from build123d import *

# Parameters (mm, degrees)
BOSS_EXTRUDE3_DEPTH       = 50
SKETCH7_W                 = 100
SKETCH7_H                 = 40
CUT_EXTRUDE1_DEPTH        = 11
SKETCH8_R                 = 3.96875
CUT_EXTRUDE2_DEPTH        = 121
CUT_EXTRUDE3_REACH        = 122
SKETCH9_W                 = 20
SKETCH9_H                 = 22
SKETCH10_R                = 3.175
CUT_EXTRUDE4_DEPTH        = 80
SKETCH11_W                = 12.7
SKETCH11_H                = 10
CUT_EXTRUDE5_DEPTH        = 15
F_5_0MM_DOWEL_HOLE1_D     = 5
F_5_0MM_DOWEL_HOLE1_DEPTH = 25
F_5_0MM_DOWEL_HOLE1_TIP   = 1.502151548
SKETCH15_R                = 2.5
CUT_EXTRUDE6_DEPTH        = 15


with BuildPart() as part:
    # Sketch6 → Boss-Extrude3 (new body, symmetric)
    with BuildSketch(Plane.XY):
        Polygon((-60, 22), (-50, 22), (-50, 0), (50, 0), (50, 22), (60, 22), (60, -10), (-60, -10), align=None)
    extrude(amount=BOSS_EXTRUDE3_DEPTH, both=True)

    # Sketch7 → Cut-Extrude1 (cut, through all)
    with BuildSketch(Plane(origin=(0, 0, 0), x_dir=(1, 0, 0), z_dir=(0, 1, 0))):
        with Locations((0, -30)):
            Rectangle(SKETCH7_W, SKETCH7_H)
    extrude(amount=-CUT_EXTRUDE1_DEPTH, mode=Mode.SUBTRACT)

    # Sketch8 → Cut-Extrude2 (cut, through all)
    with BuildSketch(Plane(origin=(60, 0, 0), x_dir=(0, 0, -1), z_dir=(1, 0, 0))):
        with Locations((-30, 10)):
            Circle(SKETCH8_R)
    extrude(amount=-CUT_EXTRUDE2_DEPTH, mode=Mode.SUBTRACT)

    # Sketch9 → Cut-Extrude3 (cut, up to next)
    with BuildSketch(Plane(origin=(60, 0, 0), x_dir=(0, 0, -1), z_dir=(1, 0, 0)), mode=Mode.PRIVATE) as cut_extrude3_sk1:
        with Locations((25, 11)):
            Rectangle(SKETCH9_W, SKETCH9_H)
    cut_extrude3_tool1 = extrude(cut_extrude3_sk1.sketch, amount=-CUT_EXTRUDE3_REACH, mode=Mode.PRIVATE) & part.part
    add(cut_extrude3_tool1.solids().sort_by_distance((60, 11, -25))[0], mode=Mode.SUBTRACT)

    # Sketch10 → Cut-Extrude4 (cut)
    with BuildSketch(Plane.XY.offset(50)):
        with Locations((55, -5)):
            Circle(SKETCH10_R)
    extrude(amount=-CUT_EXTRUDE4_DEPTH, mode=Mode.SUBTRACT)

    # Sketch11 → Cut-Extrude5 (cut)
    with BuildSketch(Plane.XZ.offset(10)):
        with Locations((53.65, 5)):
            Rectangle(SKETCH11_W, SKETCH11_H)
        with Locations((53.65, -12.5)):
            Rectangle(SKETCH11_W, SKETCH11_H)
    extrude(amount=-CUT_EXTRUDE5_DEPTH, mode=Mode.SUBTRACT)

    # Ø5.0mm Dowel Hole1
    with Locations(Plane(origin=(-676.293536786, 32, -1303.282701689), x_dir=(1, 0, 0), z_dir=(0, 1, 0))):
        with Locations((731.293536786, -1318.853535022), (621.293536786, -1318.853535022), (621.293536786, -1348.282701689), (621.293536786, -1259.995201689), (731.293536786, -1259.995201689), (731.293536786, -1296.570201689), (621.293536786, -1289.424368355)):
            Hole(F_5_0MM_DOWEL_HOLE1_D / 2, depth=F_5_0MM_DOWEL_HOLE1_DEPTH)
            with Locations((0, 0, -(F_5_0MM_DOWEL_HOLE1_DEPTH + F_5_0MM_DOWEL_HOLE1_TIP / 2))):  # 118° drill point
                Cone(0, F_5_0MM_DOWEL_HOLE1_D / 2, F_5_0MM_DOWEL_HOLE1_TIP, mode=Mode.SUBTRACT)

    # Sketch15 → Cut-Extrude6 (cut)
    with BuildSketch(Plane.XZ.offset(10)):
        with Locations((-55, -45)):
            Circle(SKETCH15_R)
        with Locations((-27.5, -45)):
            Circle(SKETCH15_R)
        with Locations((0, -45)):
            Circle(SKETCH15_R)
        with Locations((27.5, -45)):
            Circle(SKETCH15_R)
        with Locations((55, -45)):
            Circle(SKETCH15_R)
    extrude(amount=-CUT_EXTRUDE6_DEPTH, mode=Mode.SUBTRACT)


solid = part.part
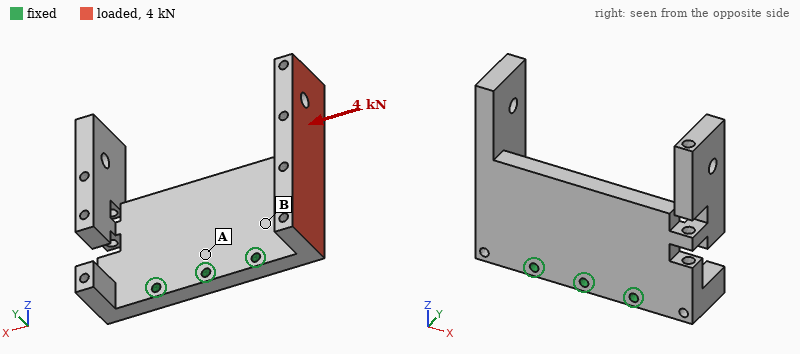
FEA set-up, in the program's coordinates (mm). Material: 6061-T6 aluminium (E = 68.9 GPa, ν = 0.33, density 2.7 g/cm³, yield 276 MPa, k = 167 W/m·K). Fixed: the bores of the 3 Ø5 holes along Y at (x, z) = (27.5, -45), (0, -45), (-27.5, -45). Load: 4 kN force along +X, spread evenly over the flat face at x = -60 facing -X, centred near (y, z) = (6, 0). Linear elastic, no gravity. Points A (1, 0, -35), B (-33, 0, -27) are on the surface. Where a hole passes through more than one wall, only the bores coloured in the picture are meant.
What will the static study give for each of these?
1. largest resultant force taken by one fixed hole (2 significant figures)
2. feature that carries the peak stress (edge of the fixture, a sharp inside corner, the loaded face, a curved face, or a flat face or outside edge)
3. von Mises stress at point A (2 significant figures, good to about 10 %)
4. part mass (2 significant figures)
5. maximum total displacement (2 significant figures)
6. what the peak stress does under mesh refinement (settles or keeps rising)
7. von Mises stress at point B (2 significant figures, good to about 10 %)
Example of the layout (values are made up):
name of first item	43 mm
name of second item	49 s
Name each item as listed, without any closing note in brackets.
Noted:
largest resultant force taken by one fixed hole	3.4 kN
feature that carries the peak stress	edge of the fixture
von Mises stress at point A	16 MPa
part mass	300 g
maximum total displacement	0.46 mm
what the peak stress does under mesh refinement	keeps rising
von Mises stress at point B	43 MPa
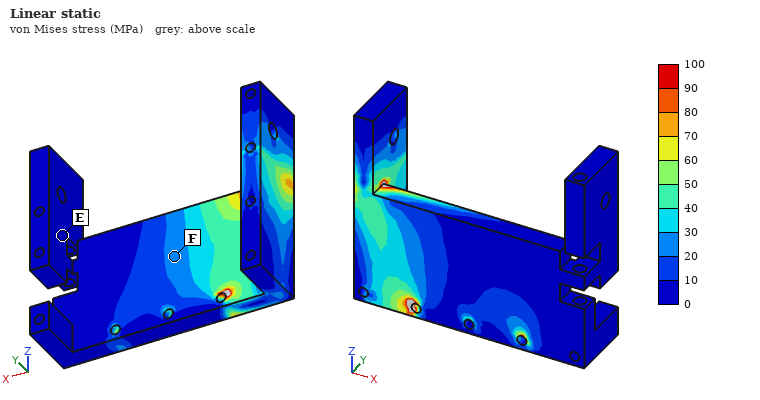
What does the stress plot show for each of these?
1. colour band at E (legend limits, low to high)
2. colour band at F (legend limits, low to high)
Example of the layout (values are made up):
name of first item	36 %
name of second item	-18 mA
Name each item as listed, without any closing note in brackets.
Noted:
colour band at E	0 to 10 MPa
colour band at F	20 to 30 MPa
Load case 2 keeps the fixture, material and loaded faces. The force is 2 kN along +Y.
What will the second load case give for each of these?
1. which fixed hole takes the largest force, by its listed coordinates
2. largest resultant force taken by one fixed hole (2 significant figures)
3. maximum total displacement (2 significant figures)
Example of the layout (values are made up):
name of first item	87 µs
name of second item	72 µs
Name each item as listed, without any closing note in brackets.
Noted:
which fixed hole takes the largest force, by its listed coordinates	(-27.5, -45)
largest resultant force taken by one fixed hole	2.8 kN
maximum total displacement	0.84 mm
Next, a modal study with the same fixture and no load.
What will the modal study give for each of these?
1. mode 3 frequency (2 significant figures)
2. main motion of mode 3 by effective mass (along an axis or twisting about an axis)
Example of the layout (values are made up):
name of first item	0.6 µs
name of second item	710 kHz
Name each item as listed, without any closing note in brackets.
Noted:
mode 3 frequency	1000 Hz
main motion of mode 3 by effective mass	along Y
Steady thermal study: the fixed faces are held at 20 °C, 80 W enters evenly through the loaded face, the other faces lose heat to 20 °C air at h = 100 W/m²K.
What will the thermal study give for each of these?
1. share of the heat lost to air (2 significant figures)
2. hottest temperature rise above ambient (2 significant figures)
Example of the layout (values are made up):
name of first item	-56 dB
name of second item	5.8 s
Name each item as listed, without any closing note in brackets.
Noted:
share of the heat lost to air	39 %
hottest temperature rise above ambient	41 K
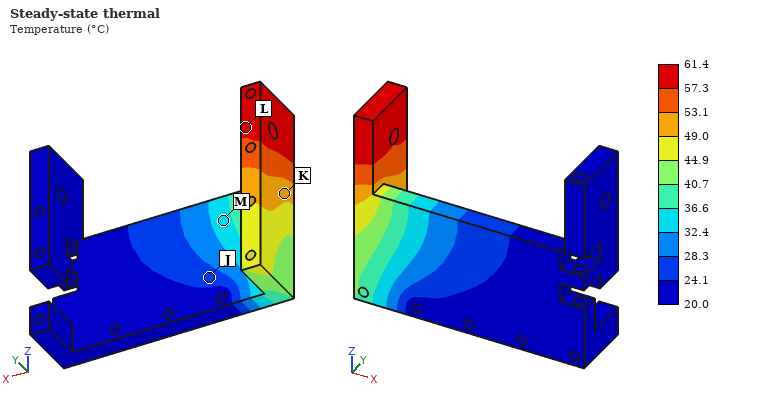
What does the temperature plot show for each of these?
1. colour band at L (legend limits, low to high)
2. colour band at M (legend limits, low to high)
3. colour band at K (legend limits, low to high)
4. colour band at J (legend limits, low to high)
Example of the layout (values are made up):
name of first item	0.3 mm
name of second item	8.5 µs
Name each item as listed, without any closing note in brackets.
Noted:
colour band at L	57.3 to 61.4 °C
colour band at M	32.4 to 36.6 °C
colour band at K	49.0 to 53.1 °C
colour band at J	24.1 to 28.3 °C
